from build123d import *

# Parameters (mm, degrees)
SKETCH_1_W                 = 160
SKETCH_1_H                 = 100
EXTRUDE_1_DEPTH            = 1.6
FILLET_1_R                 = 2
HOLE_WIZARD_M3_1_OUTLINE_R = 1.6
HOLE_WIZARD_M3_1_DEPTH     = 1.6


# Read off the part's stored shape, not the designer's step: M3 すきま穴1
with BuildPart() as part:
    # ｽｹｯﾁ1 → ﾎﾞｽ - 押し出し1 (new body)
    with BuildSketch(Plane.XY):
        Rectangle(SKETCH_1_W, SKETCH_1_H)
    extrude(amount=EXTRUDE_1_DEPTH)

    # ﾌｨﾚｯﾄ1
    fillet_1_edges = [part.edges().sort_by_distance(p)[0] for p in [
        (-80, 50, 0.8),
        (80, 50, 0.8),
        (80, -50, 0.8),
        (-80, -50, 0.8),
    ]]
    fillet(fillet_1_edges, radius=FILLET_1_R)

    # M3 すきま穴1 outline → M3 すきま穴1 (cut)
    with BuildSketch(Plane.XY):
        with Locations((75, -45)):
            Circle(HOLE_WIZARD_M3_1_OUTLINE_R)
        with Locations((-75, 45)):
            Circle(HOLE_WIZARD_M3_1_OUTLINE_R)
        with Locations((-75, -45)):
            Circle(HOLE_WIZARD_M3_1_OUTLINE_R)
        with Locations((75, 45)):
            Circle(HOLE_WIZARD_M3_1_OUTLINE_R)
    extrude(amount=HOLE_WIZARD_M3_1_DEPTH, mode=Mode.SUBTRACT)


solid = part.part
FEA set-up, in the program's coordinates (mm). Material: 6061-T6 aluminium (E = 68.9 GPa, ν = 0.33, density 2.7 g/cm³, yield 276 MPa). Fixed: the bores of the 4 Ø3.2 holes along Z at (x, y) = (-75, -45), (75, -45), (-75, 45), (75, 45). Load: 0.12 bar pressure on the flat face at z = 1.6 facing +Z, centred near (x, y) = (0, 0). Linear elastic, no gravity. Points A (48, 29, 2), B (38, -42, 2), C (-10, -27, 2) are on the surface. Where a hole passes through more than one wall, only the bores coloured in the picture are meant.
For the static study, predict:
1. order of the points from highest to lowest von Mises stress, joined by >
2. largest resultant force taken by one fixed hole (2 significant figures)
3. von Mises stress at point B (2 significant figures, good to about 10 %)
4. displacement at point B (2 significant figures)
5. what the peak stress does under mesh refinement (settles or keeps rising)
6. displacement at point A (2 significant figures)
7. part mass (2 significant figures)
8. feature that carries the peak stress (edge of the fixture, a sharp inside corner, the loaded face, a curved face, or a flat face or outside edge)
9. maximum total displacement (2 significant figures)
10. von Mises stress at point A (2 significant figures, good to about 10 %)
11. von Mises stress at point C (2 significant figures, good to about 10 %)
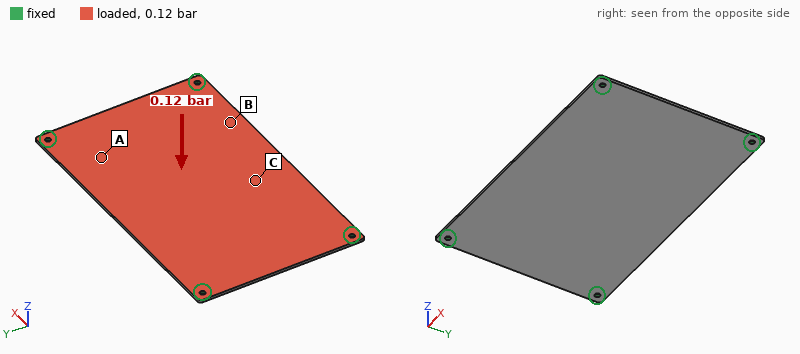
C > B > A
48 N
19 MPa
0.64 mm
keeps rising
0.50 mm
69 g
edge of the fixture
1.1 mm
11 MPa
31 MPa
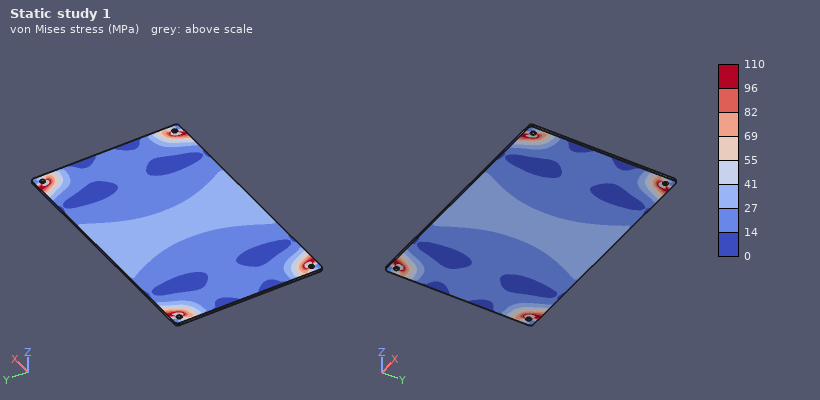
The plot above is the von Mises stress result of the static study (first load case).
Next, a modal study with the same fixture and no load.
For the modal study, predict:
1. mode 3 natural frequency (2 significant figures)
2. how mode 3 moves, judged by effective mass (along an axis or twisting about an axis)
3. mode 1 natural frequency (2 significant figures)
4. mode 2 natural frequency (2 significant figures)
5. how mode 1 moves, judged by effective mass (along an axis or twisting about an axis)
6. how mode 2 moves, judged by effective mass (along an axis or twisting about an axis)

760 Hz
twisting about Y
290 Hz
510 Hz
along Z
twisting about X
